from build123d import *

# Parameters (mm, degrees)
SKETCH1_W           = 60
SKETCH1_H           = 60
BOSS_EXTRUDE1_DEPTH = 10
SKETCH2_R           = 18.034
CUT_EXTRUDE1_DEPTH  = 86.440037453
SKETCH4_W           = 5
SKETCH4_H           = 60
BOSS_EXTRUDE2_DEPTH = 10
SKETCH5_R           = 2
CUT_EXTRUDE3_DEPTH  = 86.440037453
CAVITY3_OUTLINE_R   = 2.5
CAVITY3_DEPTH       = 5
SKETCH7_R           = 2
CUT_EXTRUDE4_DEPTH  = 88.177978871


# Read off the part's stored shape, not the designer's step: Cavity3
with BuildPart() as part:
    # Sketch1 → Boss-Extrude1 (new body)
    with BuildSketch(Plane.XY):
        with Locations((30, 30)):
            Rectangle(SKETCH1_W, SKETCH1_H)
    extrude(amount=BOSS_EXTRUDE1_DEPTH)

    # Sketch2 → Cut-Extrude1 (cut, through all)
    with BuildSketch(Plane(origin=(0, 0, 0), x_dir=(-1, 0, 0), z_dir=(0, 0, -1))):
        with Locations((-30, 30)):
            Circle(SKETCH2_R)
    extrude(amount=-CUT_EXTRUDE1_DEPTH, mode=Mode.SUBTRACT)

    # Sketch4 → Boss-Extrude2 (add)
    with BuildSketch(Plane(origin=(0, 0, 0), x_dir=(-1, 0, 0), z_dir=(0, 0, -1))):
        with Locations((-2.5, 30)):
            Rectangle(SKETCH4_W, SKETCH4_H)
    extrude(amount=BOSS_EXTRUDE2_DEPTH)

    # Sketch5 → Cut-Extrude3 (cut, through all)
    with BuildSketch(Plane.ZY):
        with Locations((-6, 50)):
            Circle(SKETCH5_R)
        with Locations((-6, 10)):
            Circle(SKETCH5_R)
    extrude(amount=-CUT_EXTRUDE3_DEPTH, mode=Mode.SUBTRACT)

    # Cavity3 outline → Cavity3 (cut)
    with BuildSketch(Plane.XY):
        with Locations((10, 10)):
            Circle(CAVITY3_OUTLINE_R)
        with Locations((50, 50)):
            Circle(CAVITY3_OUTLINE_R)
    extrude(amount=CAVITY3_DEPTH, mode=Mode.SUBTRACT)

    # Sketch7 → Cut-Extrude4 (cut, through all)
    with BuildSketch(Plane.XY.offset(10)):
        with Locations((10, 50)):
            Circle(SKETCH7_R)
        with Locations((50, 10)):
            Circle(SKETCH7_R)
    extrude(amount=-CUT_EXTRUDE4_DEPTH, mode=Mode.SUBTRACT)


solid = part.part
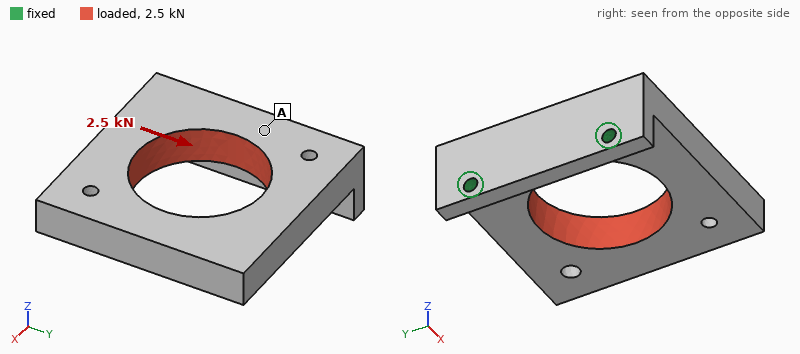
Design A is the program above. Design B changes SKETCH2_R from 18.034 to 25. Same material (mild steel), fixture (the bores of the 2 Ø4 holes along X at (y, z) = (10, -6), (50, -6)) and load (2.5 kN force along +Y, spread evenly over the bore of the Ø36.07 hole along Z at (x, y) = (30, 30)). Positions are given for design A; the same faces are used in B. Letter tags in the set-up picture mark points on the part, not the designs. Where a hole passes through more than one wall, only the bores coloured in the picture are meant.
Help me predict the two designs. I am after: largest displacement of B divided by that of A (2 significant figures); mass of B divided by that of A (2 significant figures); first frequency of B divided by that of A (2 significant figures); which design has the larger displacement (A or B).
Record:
3.1
0.67
1.1
B
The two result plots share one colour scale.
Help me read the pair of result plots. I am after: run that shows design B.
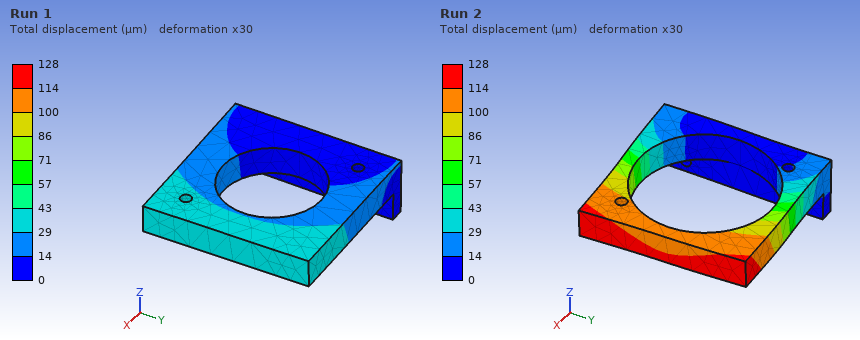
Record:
Run 2
